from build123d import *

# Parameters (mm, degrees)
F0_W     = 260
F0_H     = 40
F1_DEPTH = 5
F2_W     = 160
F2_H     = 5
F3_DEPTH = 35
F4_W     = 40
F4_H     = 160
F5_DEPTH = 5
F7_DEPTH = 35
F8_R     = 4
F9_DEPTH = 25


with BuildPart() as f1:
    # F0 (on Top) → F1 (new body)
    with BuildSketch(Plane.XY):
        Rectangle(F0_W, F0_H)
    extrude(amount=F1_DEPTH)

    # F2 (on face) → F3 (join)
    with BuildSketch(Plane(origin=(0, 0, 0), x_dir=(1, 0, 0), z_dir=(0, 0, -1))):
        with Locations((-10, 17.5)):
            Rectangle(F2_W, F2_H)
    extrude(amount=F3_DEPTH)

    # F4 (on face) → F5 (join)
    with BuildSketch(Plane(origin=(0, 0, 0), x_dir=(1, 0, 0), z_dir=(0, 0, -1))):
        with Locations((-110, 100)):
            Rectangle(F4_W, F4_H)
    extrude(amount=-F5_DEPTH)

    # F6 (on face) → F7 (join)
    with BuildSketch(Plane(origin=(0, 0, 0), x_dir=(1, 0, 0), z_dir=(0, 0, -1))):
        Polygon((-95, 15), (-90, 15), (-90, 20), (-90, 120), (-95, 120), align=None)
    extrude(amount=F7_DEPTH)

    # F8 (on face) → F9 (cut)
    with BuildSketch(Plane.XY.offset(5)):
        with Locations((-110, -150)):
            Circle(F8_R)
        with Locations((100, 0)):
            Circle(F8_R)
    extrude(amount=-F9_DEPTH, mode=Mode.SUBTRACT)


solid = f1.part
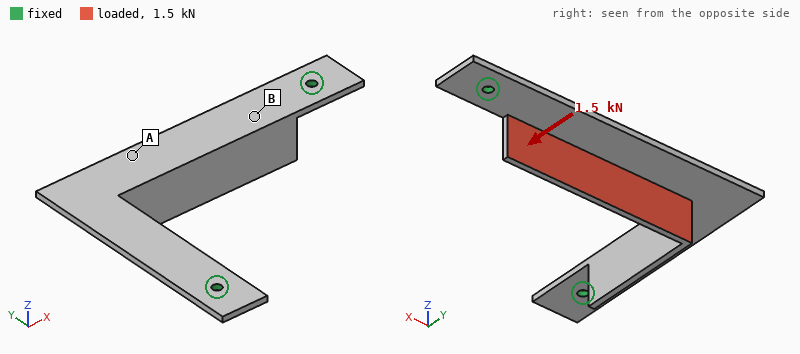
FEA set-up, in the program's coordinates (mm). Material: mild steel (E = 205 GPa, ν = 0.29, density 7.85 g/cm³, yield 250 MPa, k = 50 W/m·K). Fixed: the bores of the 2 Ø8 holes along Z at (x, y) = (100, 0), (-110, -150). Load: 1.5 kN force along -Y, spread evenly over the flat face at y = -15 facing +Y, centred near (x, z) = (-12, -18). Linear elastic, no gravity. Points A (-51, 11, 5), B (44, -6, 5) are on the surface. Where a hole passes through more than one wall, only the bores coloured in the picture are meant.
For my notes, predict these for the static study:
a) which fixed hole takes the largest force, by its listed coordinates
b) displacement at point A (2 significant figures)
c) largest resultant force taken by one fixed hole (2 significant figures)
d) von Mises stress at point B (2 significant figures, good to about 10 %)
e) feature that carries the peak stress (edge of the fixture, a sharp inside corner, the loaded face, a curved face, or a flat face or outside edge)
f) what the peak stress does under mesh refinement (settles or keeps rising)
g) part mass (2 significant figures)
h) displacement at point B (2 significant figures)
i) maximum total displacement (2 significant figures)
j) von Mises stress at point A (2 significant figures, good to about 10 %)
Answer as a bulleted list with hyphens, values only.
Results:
- (-110, -150)
- 0.43 mm
- 910 N
- 36 MPa
- edge of the fixture
- keeps rising
- 1.0 kg
- 0.100 mm
- 0.61 mm
- 11 MPa
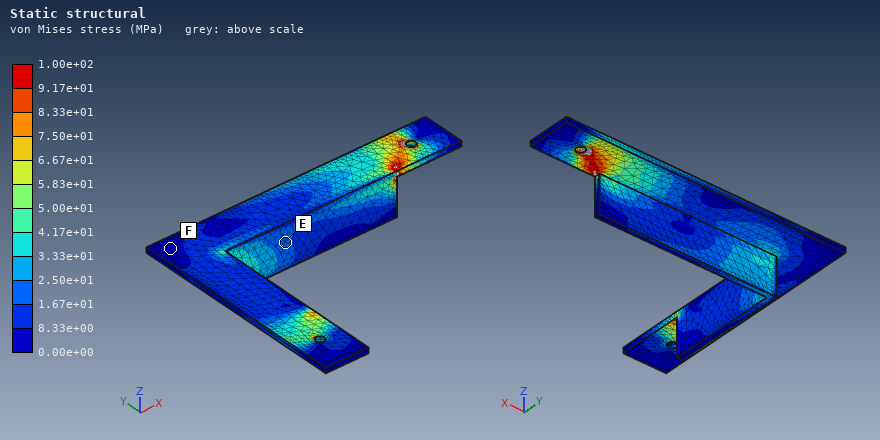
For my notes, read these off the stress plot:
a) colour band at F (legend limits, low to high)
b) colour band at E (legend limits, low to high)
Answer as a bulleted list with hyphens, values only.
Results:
- 0.00e+00 to 8.33e+00 MPa
- 1.67e+01 to 2.50e+01 MPa
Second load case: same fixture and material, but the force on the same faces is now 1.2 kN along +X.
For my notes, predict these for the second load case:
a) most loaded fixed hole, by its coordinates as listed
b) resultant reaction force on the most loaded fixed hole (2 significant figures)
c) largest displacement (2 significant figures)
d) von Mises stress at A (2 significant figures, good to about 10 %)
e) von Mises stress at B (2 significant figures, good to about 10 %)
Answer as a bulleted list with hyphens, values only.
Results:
- (100, 0)
- 1.2 kN
- 0.47 mm
- 8.2 MPa
- 9.7 MPa
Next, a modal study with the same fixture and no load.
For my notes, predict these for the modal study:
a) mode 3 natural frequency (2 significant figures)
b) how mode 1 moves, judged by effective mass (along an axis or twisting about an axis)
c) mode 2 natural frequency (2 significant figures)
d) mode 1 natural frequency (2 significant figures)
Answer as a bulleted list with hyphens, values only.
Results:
- 1200 Hz
- along Z
- 1000 Hz
- 160 Hz
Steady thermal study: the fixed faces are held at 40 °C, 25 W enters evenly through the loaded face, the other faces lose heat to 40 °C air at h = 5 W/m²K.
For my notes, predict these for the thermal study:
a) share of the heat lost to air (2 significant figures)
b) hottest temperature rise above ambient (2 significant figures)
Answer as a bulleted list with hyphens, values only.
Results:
- 41 %
- 75 K
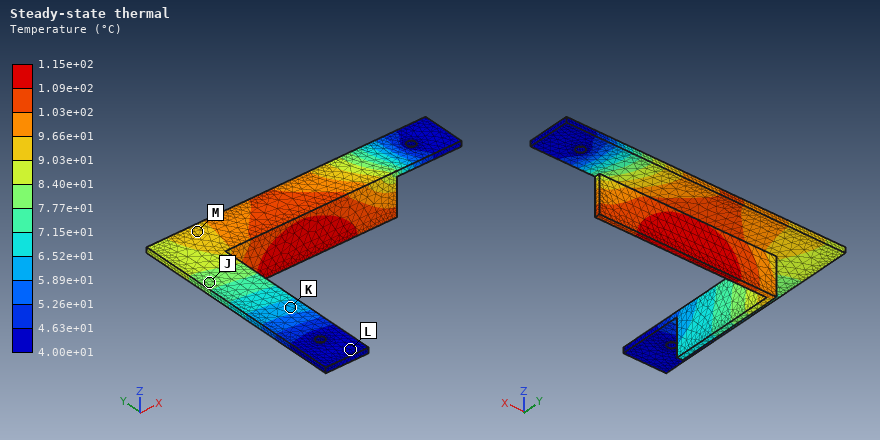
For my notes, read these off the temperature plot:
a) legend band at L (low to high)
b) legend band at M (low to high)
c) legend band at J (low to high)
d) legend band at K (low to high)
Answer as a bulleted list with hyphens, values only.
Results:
- 4.00e+01 to 4.63e+01 °C
- 9.03e+01 to 9.66e+01 °C
- 7.77e+01 to 8.40e+01 °C
- 5.89e+01 to 6.52e+01 °C
